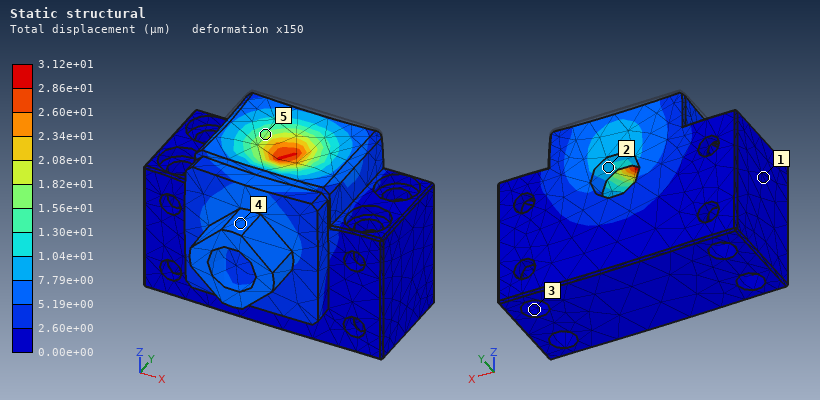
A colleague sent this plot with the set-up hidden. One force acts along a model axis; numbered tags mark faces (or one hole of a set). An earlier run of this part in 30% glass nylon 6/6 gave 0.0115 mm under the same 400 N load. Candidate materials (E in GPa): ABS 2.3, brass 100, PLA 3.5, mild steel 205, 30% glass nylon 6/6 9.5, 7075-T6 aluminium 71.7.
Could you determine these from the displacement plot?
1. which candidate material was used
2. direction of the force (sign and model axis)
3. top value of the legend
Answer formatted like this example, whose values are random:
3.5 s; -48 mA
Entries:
PLA; -Z; 3.12e+01 µm
